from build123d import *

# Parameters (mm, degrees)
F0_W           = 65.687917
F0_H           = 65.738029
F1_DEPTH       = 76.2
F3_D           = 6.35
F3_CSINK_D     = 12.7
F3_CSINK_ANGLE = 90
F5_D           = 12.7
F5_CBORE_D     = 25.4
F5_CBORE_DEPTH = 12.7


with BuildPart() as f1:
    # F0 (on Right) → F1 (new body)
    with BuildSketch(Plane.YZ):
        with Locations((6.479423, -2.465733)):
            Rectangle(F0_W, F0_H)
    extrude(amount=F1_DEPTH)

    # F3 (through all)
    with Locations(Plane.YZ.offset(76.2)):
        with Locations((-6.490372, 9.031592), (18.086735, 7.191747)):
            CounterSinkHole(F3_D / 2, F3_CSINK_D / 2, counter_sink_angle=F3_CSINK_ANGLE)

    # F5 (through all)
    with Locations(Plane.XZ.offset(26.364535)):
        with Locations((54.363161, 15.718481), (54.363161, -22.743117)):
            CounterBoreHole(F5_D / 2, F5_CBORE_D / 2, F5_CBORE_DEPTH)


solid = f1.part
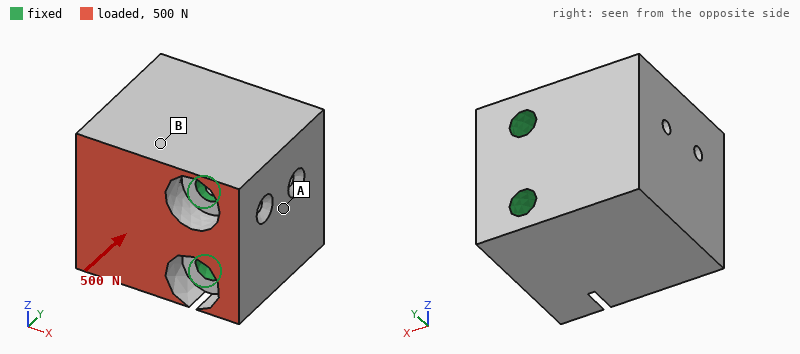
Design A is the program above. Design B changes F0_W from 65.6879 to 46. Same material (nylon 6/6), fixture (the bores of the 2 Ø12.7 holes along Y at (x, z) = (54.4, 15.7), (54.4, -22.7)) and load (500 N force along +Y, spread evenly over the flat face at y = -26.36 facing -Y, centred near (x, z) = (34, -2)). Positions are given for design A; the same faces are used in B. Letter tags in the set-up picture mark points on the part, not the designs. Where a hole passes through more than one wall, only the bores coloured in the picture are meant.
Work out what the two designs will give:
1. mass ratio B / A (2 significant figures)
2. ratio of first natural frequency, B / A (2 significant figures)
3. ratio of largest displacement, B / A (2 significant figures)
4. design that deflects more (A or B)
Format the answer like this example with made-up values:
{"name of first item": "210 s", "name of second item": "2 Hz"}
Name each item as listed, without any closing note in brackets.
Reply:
{"mass ratio B / A": "0.71", "ratio of first natural frequency, B / A": "1.0", "ratio of largest displacement, B / A": "1.4", "design that deflects more": "B"}
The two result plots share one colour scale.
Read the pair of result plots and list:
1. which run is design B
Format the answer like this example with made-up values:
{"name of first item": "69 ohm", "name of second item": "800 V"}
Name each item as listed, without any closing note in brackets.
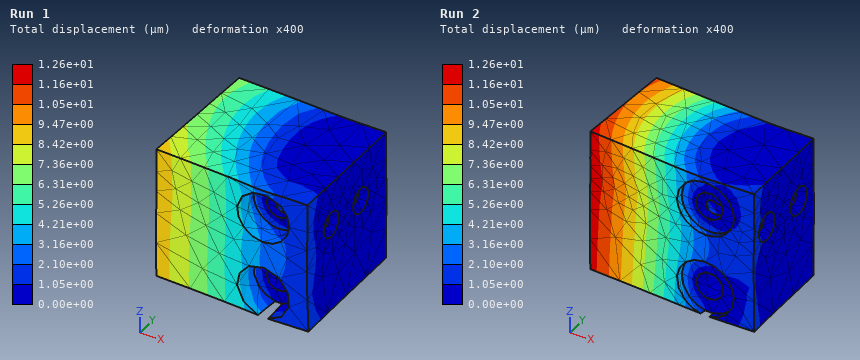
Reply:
{"which run is design B": "Run 2"}
